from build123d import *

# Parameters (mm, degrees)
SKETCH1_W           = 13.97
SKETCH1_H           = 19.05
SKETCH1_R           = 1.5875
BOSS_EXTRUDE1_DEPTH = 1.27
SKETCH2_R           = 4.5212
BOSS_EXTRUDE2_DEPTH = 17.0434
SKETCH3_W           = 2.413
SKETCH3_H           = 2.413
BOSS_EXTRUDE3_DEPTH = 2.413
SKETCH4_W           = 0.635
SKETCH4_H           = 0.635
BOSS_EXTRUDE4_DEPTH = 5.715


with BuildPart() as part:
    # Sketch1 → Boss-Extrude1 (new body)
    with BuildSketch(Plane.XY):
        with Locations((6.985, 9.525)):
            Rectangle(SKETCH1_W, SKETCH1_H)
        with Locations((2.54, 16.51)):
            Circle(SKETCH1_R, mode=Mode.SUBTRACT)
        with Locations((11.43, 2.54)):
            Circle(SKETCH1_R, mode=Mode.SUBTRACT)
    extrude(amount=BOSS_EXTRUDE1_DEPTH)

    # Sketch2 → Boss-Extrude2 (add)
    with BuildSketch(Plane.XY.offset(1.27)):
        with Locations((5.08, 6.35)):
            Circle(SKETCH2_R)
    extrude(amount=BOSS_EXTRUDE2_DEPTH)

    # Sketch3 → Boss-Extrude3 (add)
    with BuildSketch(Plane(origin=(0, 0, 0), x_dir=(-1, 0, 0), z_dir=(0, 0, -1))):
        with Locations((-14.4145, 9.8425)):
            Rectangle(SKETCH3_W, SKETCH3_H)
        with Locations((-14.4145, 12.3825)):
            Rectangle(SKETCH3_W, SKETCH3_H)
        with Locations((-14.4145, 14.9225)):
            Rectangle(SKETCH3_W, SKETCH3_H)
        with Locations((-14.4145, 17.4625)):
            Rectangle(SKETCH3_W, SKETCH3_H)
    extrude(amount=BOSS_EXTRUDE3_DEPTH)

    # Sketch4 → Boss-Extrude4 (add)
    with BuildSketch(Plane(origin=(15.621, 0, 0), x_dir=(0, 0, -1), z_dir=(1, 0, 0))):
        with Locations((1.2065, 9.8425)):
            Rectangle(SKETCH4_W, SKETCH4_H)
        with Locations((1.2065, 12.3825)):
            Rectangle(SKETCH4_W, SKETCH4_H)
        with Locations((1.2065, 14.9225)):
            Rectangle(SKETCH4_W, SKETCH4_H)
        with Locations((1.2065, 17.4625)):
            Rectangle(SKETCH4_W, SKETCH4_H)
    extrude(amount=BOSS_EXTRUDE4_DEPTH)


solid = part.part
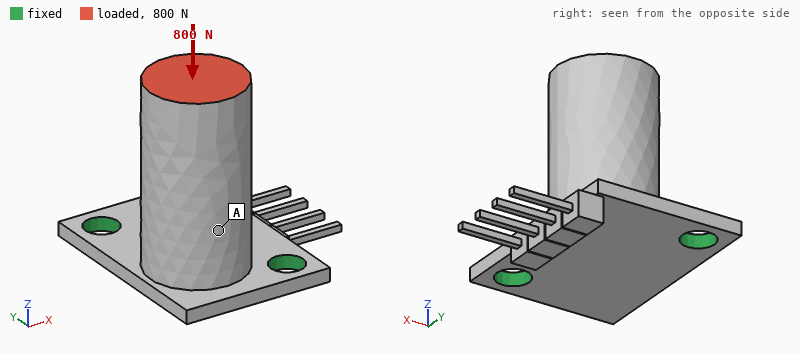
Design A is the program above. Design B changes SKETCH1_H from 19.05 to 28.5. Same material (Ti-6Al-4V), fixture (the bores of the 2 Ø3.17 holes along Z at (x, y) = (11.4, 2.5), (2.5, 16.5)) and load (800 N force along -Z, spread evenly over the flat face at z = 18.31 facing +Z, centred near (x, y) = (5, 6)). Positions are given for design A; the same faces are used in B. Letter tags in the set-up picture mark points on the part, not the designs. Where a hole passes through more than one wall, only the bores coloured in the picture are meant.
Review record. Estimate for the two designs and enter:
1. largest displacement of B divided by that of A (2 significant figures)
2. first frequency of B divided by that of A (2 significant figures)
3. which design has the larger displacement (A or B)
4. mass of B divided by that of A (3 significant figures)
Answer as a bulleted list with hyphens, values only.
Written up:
- 0.89
- 1.1
- A
- 1.11
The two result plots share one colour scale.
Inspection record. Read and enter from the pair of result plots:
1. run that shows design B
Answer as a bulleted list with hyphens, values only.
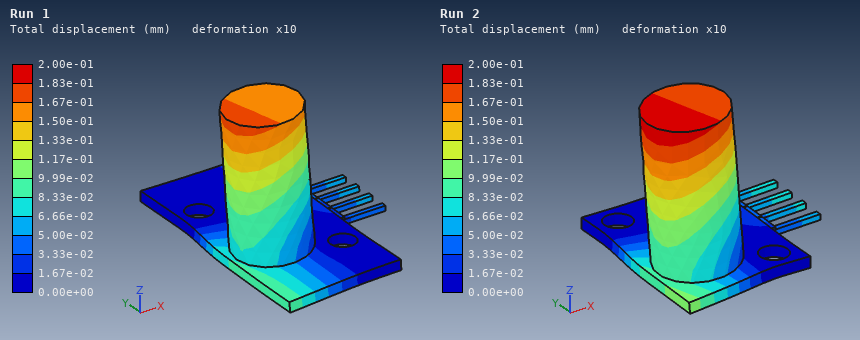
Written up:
- Run 1
